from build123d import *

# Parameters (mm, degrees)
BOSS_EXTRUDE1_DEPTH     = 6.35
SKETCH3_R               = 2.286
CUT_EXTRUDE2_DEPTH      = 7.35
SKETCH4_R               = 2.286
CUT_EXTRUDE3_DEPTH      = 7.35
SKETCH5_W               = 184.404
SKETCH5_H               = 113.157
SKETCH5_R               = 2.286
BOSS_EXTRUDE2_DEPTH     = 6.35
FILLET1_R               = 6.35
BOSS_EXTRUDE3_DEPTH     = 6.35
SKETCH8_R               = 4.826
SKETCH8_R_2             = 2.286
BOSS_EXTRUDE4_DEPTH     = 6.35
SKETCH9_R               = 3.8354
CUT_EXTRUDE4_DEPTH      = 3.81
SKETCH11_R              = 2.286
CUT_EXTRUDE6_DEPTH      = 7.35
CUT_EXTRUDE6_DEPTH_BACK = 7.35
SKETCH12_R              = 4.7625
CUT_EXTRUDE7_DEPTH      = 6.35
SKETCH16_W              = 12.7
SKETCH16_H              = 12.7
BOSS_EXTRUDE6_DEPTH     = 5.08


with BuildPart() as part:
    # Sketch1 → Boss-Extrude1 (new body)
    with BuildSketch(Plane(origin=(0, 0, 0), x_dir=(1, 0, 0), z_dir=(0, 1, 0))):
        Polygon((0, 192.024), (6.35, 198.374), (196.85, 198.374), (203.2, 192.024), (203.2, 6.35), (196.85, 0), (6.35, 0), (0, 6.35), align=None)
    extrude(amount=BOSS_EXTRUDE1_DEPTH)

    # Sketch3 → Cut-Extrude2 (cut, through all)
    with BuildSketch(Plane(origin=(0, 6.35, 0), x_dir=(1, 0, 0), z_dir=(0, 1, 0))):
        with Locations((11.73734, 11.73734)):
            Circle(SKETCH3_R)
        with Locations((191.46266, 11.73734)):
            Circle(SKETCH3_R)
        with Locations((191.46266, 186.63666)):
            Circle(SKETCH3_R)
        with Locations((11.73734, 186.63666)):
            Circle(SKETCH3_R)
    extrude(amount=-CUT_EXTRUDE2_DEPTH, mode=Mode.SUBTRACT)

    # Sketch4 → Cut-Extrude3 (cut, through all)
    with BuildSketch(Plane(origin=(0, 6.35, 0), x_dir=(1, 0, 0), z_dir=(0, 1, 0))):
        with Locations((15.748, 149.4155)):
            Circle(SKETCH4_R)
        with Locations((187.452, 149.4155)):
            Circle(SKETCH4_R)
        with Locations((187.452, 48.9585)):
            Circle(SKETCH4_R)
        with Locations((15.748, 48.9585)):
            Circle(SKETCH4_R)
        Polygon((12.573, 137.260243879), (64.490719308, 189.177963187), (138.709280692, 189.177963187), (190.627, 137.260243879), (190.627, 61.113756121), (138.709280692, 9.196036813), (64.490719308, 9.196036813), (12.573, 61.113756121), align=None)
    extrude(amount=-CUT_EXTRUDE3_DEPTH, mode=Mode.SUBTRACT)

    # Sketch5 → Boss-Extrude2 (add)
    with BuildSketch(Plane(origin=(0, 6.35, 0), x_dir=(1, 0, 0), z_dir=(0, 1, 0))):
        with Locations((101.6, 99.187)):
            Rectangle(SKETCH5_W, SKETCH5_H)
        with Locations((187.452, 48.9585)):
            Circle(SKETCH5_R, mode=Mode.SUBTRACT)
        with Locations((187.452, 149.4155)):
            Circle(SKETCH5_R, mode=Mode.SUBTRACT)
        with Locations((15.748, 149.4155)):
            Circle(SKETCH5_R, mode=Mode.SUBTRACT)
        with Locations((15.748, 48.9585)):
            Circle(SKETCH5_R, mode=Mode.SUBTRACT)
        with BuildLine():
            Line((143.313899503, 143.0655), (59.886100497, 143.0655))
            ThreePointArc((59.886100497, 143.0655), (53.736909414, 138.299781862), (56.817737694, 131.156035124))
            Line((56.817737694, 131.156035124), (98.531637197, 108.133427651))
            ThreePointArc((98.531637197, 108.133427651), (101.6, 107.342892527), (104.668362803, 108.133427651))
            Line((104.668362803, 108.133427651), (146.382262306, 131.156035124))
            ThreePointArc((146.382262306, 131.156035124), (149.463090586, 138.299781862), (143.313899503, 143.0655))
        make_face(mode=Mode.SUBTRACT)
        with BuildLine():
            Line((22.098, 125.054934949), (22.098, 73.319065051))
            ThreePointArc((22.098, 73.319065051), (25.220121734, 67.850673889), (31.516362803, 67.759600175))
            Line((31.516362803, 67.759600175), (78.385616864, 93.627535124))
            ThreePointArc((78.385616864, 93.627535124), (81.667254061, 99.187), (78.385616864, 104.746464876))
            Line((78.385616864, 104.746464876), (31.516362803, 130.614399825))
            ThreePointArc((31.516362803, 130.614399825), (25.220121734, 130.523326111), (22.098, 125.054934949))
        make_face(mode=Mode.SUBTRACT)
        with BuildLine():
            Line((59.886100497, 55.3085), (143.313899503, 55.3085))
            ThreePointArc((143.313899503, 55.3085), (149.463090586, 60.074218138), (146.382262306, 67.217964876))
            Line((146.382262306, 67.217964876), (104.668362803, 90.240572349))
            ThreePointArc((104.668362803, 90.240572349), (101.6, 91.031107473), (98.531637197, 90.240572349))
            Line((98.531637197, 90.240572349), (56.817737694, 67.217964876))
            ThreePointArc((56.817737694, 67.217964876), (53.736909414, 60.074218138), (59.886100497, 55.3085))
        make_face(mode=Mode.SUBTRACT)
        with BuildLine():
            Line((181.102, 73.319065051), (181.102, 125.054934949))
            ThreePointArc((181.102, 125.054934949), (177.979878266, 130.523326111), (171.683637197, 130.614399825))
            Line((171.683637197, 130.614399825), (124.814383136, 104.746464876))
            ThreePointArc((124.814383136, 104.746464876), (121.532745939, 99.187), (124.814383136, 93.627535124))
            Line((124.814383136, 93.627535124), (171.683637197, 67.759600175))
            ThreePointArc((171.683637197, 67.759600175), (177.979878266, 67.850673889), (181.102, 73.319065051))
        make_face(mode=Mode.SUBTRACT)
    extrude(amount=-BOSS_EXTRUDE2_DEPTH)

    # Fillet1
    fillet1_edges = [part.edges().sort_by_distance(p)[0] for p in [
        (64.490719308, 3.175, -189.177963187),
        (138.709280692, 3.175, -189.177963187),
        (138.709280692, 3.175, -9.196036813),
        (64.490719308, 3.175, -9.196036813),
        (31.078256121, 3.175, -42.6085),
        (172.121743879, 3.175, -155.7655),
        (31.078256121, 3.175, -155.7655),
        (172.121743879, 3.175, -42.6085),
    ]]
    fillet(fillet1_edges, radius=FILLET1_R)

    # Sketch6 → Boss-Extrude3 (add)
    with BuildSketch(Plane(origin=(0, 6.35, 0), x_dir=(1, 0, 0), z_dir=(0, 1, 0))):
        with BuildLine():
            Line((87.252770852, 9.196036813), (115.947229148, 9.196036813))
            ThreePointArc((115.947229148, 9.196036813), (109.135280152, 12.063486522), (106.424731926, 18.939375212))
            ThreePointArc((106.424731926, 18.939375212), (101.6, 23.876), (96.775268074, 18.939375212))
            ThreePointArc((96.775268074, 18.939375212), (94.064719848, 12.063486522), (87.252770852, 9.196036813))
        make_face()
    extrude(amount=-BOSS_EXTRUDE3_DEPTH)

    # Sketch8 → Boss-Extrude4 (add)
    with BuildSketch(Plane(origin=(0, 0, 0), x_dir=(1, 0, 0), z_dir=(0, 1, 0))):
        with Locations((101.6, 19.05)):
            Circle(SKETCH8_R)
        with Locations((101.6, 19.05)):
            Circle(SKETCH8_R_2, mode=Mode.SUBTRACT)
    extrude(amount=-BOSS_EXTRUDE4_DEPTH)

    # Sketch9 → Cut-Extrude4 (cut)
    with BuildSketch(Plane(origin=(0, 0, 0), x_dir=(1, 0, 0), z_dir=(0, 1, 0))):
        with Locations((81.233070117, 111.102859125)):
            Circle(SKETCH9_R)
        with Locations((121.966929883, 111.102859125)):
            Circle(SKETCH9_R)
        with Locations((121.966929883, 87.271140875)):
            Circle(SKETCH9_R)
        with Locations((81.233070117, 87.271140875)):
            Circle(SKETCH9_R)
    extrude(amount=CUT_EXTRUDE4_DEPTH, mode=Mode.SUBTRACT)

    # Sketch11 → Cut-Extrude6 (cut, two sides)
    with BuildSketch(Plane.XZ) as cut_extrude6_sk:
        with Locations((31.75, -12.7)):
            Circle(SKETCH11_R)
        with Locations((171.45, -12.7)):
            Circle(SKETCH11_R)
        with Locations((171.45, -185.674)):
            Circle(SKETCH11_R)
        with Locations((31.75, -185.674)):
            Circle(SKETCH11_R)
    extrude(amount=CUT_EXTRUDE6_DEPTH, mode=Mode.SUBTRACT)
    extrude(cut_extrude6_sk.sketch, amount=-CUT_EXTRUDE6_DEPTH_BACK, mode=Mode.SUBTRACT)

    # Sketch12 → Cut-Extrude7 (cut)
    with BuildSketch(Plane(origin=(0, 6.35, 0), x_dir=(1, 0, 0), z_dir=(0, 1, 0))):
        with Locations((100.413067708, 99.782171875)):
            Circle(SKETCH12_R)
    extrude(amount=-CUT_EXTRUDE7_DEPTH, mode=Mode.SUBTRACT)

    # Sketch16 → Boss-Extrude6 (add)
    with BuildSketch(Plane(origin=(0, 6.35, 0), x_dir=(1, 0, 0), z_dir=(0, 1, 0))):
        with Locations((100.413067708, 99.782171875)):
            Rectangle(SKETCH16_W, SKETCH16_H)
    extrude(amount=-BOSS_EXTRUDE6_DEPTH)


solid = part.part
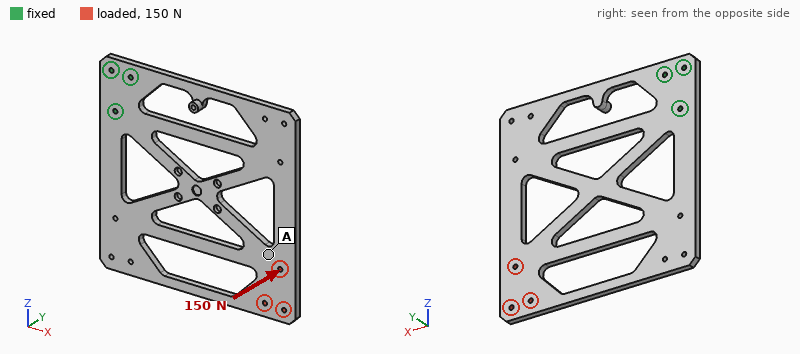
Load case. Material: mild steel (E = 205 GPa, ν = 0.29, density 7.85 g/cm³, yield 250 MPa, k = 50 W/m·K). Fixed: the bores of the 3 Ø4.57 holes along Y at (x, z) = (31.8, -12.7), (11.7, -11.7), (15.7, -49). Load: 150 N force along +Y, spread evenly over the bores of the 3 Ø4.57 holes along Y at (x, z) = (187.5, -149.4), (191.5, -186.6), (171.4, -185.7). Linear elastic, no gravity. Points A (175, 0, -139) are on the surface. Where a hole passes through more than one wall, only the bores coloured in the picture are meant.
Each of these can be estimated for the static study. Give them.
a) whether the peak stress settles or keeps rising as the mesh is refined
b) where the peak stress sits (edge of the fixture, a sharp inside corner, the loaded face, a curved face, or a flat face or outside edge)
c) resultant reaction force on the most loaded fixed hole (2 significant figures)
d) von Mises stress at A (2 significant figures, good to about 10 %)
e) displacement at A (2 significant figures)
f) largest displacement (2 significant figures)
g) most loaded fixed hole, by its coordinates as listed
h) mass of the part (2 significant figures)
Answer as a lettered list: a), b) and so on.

a) keeps rising
b) edge of the fixture
c) 350 N
d) 10 MPa
e) 1.5 mm
f) 2.3 mm
g) (15.7, -49)
h) 1.2 kg
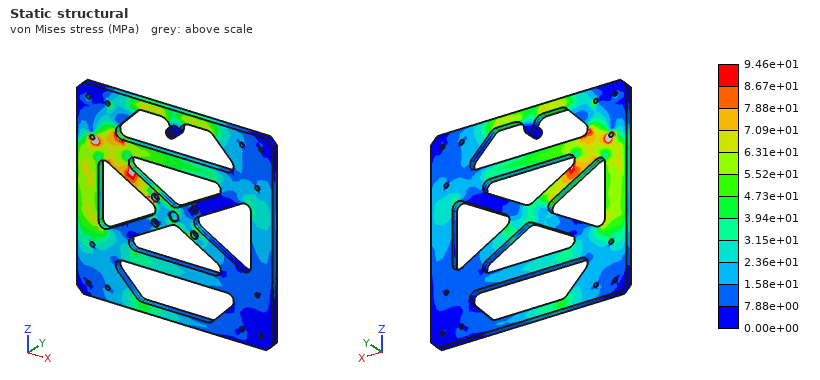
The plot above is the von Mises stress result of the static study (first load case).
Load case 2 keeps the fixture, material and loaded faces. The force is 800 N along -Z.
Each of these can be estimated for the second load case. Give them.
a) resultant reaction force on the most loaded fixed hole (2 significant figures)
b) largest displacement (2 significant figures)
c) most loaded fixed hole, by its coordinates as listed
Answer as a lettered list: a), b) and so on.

a) 2.7 kN
b) 0.19 mm
c) (15.7, -49)
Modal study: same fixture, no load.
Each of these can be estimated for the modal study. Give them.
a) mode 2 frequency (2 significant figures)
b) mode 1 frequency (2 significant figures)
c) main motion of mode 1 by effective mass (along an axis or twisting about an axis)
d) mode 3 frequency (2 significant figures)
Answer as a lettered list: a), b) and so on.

a) 170 Hz
b) 82 Hz
c) along Y
d) 330 Hz
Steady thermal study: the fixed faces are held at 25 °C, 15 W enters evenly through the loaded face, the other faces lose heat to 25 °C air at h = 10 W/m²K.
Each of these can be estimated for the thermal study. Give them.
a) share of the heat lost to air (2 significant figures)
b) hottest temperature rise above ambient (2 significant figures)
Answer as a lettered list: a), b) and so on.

a) 87 %
b) 76 K
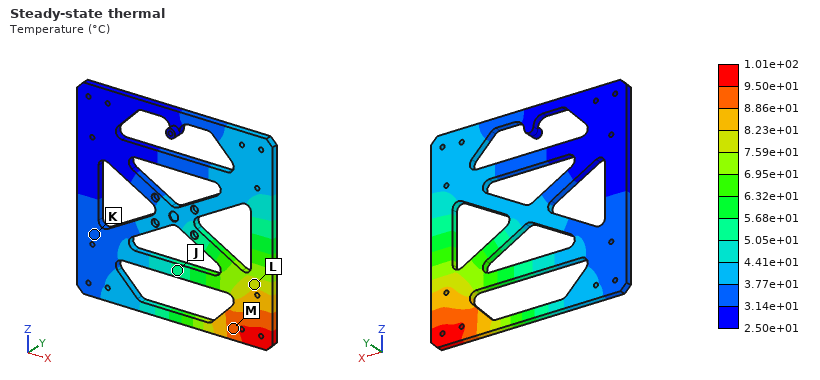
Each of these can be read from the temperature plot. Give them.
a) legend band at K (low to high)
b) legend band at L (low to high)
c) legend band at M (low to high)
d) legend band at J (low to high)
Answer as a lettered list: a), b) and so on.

a) 3.14e+01 to 3.77e+01 °C
b) 7.59e+01 to 8.23e+01 °C
c) 8.86e+01 to 9.50e+01 °C
d) 5.05e+01 to 5.68e+01 °C
